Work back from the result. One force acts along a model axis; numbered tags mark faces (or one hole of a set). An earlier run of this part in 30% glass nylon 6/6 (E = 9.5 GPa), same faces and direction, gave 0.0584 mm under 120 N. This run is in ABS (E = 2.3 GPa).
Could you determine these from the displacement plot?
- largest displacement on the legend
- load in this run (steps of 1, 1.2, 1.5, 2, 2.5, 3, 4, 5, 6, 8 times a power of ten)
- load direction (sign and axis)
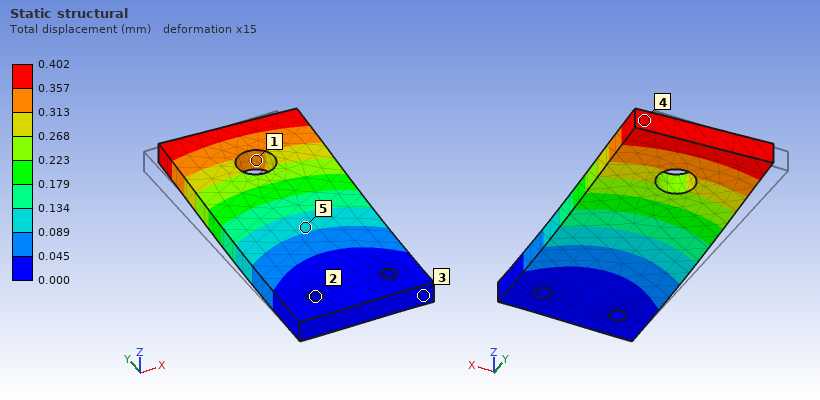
0.402 mm
200 N
+X
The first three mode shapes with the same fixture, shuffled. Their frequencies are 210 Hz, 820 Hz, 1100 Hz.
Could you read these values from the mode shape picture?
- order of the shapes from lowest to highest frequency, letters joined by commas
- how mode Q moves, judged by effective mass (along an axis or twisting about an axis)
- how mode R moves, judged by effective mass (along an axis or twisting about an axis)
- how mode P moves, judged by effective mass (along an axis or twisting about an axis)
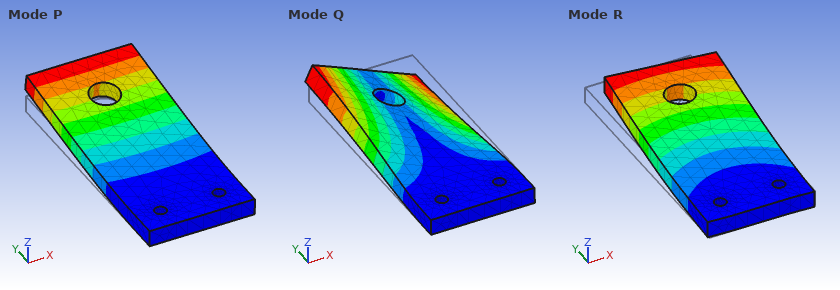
P, Q, R
twisting about Y
along X
along Z
